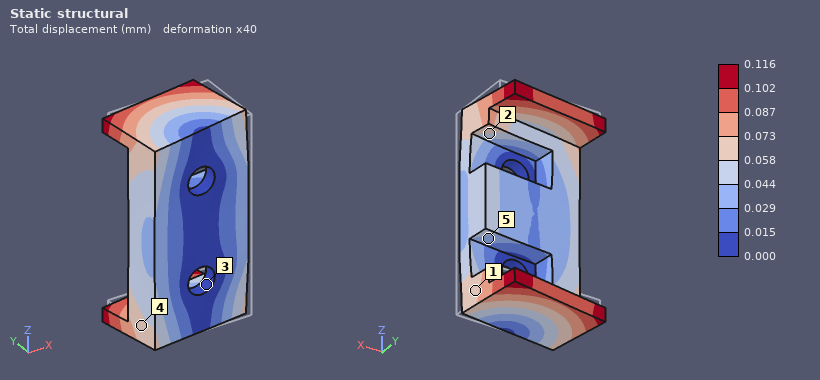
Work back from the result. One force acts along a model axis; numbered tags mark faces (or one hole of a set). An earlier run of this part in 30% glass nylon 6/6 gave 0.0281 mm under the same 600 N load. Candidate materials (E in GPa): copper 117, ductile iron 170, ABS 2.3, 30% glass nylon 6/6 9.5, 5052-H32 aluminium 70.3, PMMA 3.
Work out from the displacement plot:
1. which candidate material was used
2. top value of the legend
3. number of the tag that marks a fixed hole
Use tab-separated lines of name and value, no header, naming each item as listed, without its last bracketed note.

which candidate material was used	ABS
top value of the legend	0.116 mm
number of the tag that marks a fixed hole	3
